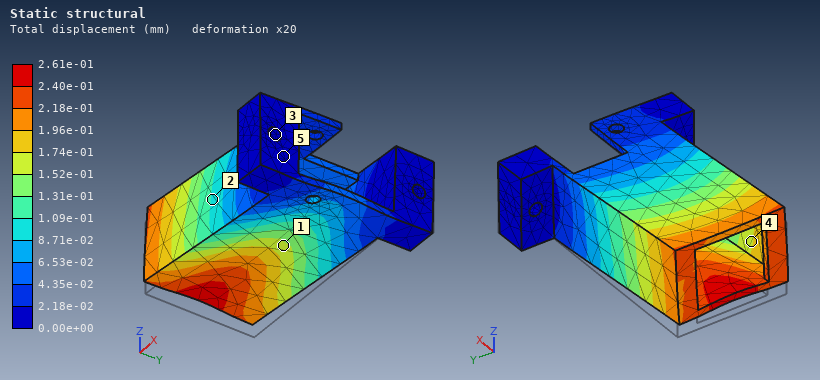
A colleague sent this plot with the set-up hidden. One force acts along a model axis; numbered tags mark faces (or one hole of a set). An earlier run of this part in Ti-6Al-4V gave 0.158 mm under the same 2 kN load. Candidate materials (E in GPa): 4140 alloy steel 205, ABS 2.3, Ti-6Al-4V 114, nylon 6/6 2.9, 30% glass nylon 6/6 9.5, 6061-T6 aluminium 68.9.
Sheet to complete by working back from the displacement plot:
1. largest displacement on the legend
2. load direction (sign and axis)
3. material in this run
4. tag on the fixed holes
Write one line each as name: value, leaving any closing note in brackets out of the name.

largest displacement on the legend: 2.61e-01 mm
load direction: +Z
material in this run: 6061-T6 aluminium
tag on the fixed holes: 3
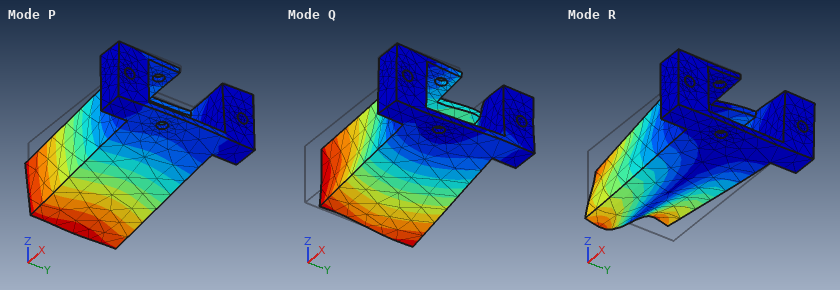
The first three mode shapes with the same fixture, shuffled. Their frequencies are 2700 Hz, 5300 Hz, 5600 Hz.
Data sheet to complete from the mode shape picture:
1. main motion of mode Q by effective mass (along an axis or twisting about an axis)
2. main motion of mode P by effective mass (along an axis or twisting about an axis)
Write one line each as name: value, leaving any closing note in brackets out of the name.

main motion of mode Q by effective mass: along Y
main motion of mode P by effective mass: along Z
